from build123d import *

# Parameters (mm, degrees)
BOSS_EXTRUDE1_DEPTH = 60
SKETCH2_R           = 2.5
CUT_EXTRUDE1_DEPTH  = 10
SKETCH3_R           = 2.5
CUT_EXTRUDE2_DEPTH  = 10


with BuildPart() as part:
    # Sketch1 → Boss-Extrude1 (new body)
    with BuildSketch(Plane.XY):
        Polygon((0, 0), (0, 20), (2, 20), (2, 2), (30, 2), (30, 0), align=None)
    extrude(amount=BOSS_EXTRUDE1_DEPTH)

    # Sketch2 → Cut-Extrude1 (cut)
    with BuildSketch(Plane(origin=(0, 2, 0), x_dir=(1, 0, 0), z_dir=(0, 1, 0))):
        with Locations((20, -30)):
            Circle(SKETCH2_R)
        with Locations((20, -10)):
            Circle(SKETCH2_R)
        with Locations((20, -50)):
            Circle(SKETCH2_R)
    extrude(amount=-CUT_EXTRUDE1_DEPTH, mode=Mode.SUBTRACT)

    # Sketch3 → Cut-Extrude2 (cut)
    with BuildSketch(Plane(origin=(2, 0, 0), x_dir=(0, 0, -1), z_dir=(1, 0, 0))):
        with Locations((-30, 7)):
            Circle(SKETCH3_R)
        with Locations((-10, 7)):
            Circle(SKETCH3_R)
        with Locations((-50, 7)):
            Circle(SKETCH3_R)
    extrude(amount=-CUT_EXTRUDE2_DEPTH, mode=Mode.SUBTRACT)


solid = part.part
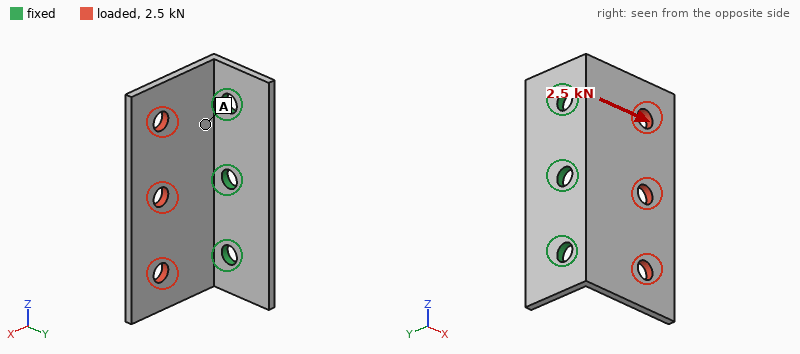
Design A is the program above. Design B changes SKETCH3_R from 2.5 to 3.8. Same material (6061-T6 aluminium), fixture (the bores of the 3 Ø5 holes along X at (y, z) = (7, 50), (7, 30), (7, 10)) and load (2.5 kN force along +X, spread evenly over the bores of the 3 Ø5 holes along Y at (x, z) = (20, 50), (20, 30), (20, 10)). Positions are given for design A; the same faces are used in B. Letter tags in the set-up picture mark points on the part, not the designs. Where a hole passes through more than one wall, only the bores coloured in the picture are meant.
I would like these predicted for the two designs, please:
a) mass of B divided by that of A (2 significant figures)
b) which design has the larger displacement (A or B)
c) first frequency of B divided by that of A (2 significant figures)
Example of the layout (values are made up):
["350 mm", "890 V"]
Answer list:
["0.97", "A", "1.1"]
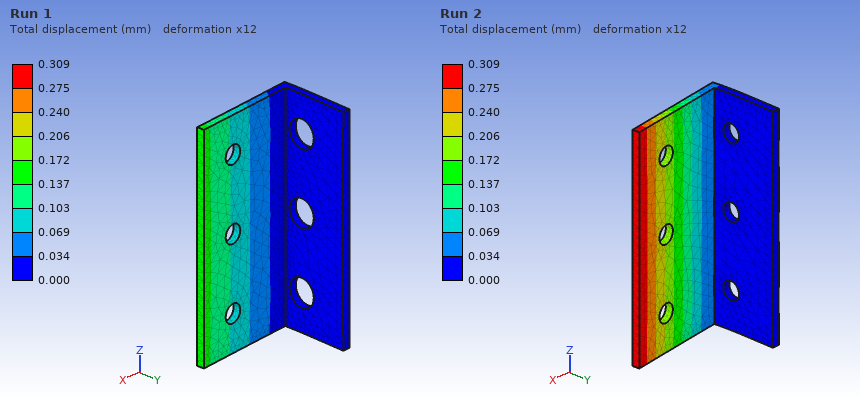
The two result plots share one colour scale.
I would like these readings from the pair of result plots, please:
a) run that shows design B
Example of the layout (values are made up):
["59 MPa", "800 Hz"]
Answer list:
["Run 1"]
